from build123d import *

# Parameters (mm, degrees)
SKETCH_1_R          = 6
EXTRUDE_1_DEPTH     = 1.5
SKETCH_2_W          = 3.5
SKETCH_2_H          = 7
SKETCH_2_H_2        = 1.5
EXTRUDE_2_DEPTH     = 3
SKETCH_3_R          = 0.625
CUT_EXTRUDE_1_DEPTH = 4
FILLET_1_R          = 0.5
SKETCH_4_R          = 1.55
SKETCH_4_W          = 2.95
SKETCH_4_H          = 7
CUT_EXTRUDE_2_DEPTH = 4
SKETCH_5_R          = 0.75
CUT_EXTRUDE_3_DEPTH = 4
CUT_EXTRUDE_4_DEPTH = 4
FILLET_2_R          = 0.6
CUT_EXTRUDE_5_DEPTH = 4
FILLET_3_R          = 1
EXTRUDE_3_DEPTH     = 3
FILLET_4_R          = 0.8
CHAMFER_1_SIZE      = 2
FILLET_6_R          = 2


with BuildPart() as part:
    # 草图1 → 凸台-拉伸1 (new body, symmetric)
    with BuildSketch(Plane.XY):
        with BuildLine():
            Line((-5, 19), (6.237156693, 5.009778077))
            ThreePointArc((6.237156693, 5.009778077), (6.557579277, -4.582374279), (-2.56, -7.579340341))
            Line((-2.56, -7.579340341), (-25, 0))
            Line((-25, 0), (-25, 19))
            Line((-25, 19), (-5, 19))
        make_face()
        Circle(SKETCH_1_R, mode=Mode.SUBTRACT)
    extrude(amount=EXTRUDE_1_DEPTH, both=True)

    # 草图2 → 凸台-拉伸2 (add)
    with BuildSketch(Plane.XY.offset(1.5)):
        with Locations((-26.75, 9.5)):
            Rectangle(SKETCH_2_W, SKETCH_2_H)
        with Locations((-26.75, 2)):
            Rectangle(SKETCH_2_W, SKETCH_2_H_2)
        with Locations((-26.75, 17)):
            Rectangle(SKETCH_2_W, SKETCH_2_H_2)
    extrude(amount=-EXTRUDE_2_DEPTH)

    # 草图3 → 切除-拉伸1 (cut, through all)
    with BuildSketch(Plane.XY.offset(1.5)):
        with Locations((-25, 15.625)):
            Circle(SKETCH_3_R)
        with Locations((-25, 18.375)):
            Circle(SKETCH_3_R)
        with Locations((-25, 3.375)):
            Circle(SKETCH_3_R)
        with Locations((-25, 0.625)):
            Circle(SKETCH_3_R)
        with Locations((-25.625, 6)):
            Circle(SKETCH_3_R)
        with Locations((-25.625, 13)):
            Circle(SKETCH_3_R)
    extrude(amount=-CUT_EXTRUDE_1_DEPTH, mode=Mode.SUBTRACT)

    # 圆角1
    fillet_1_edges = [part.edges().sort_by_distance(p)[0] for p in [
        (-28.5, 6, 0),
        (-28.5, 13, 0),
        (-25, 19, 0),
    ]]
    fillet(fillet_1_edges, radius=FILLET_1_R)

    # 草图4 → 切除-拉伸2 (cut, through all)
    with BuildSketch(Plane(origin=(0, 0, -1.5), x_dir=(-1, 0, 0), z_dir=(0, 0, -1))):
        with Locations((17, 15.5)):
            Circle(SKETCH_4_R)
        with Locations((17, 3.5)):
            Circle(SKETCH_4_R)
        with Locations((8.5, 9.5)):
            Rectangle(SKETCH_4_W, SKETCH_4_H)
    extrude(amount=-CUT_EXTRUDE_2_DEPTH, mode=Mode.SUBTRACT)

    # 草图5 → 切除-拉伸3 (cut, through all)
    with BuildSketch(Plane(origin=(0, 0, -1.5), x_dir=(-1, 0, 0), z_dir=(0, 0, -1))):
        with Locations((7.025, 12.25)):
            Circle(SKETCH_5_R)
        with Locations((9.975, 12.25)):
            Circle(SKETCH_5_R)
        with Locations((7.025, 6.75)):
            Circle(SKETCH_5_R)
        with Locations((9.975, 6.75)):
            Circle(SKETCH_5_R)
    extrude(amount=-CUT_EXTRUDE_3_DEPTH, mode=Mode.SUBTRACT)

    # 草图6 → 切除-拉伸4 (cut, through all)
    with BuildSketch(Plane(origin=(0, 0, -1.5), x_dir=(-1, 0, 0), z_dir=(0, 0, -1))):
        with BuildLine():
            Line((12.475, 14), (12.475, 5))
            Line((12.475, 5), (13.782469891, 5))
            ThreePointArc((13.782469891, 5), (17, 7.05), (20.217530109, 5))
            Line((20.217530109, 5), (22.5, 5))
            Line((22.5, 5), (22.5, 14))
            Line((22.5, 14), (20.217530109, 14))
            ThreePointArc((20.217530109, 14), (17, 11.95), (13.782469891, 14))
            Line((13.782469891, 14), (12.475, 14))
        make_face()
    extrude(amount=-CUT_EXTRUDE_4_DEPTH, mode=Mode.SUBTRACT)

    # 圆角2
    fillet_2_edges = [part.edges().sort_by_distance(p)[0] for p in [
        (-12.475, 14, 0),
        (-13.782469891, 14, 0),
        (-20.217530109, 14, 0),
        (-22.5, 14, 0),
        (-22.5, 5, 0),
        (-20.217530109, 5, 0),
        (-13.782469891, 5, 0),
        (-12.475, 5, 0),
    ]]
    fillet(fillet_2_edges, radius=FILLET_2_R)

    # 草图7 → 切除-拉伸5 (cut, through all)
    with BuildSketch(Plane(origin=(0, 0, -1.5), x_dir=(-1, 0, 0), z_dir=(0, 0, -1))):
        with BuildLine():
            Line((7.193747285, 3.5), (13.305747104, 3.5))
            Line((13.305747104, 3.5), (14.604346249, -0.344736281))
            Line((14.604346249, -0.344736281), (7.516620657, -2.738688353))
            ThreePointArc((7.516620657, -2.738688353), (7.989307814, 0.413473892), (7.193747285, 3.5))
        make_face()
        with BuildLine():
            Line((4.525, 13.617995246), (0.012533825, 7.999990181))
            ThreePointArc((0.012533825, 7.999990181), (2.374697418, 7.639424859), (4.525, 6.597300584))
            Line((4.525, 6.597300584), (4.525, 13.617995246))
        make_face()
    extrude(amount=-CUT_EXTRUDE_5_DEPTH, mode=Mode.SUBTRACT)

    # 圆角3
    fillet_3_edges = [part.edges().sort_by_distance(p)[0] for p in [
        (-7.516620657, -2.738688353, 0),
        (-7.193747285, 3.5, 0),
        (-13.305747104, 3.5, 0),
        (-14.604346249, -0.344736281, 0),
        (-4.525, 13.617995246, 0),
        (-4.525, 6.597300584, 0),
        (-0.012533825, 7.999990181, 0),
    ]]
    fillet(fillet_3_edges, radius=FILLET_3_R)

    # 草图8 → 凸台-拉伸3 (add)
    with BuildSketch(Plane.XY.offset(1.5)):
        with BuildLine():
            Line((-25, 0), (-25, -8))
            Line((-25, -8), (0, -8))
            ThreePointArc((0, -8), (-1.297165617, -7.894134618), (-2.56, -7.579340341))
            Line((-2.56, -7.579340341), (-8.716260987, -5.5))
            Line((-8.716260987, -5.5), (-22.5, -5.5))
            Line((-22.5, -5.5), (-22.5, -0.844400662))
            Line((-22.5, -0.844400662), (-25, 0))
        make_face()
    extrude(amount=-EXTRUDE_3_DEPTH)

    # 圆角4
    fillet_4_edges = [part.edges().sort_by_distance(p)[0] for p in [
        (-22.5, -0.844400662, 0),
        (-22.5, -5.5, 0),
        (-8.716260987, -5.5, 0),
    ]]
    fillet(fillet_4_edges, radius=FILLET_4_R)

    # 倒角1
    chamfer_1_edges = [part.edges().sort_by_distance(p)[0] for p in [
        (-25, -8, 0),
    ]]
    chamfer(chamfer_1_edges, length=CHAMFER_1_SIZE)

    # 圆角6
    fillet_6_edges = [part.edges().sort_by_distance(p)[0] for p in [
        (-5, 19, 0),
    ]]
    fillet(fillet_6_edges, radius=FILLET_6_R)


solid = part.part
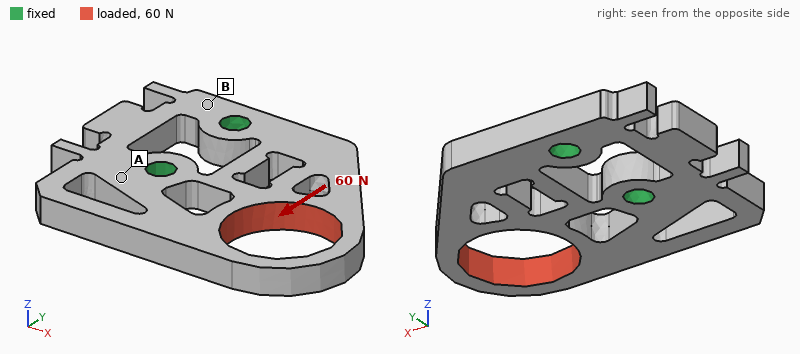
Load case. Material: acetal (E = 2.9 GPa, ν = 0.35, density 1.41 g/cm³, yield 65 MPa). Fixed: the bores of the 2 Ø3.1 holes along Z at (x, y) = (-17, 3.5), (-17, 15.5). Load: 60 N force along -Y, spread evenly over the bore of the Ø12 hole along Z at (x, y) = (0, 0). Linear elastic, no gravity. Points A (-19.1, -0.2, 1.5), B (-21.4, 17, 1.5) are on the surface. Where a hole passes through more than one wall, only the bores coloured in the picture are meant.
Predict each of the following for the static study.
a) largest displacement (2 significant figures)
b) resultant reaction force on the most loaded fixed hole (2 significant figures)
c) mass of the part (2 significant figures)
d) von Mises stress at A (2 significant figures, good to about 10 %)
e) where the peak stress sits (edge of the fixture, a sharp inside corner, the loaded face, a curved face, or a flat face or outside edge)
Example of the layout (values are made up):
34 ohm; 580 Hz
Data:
0.20 mm; 57 N; 2.1 g; 3.1 MPa; a curved face
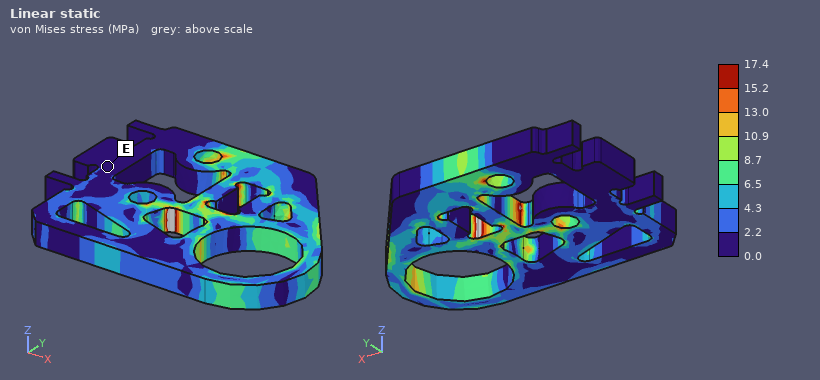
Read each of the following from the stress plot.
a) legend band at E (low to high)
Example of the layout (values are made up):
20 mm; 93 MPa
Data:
0.0 to 2.2 MPa
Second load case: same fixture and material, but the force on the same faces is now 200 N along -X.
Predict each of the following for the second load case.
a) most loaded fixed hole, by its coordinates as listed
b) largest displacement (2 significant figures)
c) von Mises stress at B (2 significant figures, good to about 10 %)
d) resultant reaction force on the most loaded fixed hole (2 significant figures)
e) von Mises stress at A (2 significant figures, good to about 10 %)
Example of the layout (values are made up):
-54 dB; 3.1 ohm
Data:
(-17, 3.5); 0.29 mm; 2.2 MPa; 200 N; 7.9 MPa
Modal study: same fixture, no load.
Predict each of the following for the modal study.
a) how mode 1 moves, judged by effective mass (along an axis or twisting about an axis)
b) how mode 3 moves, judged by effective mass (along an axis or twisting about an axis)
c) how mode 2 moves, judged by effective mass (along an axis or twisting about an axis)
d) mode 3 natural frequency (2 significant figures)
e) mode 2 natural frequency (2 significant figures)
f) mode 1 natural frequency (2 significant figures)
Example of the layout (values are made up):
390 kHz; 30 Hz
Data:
along Z; along Y; twisting about X; 3900 Hz; 2600 Hz; 1300 Hz
